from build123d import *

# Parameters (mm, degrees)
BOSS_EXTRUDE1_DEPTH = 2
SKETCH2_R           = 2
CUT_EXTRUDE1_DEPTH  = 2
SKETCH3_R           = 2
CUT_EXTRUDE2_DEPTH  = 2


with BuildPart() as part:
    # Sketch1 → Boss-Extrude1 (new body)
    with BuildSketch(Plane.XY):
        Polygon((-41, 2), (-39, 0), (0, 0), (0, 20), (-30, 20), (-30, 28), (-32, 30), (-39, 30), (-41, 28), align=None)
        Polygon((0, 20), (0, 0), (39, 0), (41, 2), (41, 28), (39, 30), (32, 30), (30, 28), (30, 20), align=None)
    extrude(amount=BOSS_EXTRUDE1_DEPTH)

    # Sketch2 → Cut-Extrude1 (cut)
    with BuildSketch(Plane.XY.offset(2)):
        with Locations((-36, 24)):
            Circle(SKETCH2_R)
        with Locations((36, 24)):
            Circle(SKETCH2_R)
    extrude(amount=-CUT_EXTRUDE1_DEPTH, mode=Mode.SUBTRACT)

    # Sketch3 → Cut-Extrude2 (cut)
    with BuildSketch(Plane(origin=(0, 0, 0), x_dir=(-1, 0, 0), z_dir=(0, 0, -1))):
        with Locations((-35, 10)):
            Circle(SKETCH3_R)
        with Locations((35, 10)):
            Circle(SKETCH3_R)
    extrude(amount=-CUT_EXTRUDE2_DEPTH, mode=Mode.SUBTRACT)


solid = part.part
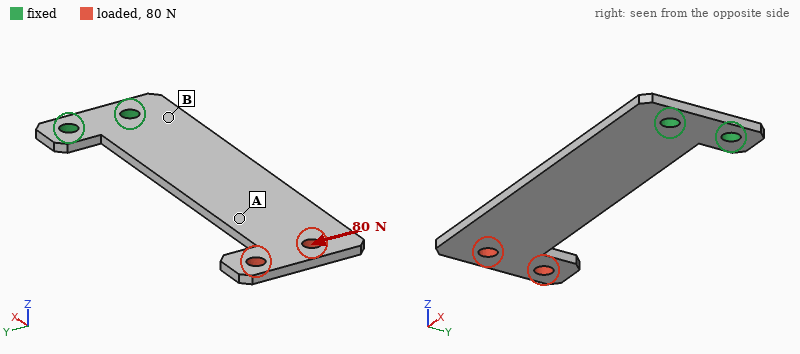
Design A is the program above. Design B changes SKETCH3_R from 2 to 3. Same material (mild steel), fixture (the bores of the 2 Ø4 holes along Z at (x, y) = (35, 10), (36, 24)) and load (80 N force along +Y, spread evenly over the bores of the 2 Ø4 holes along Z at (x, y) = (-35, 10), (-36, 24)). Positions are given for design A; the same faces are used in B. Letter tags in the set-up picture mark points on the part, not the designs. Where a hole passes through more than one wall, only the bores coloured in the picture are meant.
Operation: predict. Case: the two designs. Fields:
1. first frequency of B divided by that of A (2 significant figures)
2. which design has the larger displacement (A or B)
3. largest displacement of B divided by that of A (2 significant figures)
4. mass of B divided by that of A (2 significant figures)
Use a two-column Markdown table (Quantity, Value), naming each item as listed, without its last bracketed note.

| Quantity | Value |
|---|---|
| first frequency of B divided by that of A | 1.0 |
| which design has the larger displacement | A |
| largest displacement of B divided by that of A | 0.92 |
| mass of B divided by that of A | 0.98 |
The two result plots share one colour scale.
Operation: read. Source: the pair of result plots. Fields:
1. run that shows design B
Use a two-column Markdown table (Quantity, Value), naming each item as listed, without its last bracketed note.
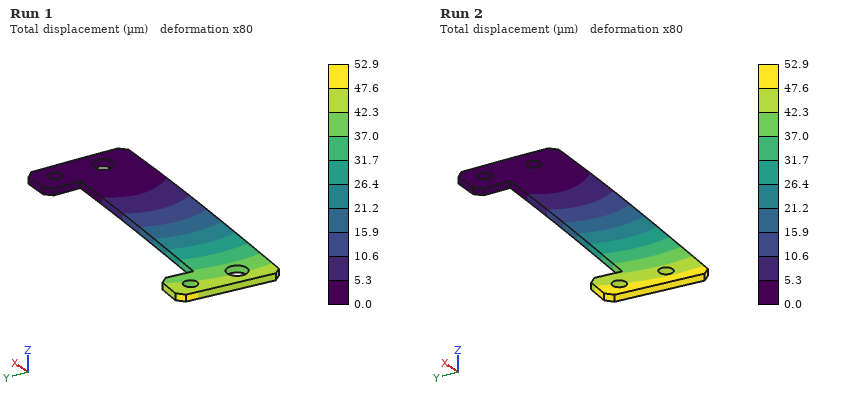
| Quantity | Value |
|---|---|
| run that shows design B | Run 1 |
